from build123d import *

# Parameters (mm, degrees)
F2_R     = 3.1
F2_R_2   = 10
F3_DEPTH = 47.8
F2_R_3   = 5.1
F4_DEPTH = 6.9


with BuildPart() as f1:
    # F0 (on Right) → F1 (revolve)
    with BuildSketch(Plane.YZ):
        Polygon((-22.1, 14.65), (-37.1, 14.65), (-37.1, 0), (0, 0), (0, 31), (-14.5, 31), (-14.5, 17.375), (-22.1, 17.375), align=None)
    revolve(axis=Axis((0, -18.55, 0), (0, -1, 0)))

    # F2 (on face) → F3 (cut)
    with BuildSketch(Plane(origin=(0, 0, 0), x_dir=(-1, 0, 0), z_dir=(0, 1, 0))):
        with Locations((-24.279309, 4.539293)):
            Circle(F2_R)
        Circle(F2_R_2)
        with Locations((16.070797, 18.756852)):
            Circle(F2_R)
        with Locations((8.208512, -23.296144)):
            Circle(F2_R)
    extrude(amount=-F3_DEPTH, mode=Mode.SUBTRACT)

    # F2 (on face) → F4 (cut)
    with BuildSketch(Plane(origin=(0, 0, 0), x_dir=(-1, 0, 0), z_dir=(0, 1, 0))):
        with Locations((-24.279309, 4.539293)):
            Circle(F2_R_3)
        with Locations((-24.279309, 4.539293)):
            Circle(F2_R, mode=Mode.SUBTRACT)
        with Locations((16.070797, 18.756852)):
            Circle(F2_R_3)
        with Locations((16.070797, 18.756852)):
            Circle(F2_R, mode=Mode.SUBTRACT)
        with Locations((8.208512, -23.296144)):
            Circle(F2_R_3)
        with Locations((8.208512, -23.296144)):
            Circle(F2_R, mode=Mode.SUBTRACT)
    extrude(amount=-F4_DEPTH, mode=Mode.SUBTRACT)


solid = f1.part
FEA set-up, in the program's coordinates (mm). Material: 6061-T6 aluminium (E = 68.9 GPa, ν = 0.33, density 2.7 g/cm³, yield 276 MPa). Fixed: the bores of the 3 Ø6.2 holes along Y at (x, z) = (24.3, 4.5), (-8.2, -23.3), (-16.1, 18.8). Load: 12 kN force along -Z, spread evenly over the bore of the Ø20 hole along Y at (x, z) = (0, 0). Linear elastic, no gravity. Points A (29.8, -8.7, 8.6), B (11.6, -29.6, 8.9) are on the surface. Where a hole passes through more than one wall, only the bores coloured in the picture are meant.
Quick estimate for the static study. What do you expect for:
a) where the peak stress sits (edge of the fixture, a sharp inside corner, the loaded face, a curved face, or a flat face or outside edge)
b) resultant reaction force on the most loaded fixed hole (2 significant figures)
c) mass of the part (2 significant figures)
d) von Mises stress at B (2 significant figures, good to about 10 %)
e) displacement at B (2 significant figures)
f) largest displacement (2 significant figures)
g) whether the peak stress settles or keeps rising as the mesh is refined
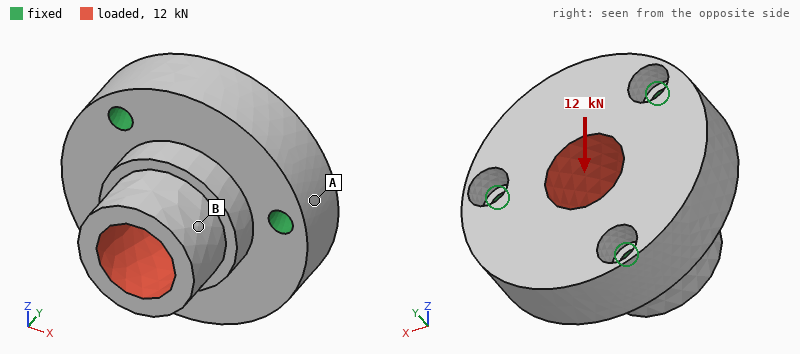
edge of the fixture
4.4 kN
130 g
17 MPa
25 µm
34 µm
keeps rising
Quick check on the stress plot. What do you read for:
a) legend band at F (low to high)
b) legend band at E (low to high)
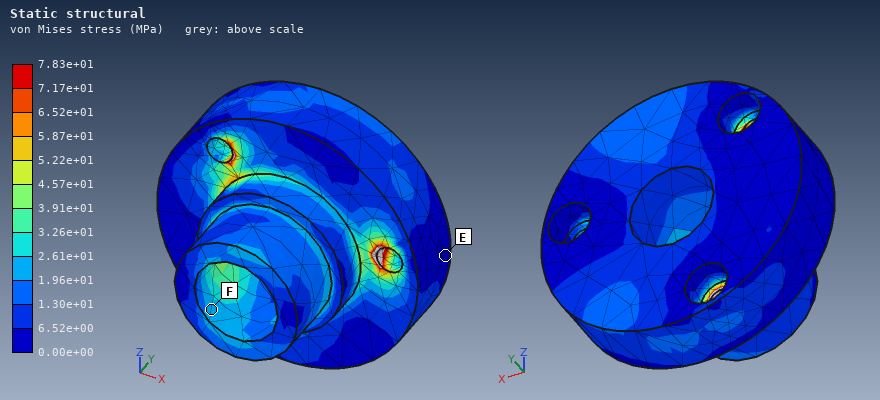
1.96e+01 to 2.61e+01 MPa
0.00e+00 to 6.52e+00 MPa
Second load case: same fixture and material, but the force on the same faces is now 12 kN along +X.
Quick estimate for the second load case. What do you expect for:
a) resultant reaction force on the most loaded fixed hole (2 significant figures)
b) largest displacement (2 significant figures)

4.4 kN
34 µm
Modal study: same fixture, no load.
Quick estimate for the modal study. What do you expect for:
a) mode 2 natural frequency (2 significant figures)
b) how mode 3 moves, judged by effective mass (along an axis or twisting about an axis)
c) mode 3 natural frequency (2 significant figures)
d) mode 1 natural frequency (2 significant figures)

14 kHz
along Y
17 kHz
14 kHz
